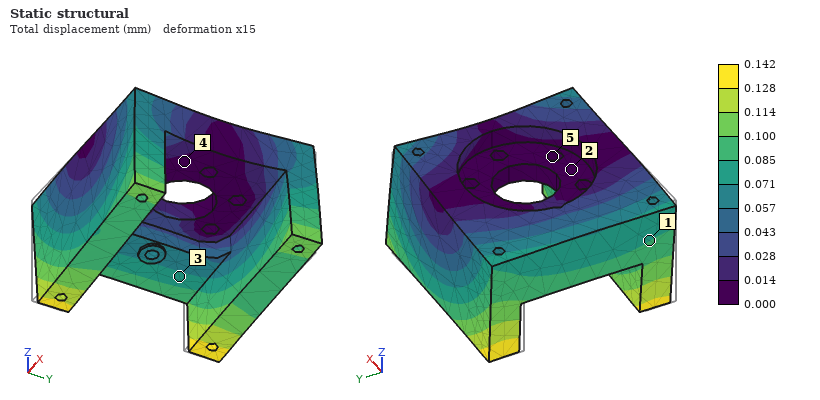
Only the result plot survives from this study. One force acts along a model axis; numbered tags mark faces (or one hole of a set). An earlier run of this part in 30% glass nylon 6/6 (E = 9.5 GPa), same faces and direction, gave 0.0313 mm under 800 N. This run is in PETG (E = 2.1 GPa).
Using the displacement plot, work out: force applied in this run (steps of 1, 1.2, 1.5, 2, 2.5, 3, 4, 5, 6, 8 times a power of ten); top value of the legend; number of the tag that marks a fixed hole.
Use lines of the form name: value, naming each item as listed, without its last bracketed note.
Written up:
force applied in this run: 800 N
top value of the legend: 0.142 mm
number of the tag that marks a fixed hole: 5
